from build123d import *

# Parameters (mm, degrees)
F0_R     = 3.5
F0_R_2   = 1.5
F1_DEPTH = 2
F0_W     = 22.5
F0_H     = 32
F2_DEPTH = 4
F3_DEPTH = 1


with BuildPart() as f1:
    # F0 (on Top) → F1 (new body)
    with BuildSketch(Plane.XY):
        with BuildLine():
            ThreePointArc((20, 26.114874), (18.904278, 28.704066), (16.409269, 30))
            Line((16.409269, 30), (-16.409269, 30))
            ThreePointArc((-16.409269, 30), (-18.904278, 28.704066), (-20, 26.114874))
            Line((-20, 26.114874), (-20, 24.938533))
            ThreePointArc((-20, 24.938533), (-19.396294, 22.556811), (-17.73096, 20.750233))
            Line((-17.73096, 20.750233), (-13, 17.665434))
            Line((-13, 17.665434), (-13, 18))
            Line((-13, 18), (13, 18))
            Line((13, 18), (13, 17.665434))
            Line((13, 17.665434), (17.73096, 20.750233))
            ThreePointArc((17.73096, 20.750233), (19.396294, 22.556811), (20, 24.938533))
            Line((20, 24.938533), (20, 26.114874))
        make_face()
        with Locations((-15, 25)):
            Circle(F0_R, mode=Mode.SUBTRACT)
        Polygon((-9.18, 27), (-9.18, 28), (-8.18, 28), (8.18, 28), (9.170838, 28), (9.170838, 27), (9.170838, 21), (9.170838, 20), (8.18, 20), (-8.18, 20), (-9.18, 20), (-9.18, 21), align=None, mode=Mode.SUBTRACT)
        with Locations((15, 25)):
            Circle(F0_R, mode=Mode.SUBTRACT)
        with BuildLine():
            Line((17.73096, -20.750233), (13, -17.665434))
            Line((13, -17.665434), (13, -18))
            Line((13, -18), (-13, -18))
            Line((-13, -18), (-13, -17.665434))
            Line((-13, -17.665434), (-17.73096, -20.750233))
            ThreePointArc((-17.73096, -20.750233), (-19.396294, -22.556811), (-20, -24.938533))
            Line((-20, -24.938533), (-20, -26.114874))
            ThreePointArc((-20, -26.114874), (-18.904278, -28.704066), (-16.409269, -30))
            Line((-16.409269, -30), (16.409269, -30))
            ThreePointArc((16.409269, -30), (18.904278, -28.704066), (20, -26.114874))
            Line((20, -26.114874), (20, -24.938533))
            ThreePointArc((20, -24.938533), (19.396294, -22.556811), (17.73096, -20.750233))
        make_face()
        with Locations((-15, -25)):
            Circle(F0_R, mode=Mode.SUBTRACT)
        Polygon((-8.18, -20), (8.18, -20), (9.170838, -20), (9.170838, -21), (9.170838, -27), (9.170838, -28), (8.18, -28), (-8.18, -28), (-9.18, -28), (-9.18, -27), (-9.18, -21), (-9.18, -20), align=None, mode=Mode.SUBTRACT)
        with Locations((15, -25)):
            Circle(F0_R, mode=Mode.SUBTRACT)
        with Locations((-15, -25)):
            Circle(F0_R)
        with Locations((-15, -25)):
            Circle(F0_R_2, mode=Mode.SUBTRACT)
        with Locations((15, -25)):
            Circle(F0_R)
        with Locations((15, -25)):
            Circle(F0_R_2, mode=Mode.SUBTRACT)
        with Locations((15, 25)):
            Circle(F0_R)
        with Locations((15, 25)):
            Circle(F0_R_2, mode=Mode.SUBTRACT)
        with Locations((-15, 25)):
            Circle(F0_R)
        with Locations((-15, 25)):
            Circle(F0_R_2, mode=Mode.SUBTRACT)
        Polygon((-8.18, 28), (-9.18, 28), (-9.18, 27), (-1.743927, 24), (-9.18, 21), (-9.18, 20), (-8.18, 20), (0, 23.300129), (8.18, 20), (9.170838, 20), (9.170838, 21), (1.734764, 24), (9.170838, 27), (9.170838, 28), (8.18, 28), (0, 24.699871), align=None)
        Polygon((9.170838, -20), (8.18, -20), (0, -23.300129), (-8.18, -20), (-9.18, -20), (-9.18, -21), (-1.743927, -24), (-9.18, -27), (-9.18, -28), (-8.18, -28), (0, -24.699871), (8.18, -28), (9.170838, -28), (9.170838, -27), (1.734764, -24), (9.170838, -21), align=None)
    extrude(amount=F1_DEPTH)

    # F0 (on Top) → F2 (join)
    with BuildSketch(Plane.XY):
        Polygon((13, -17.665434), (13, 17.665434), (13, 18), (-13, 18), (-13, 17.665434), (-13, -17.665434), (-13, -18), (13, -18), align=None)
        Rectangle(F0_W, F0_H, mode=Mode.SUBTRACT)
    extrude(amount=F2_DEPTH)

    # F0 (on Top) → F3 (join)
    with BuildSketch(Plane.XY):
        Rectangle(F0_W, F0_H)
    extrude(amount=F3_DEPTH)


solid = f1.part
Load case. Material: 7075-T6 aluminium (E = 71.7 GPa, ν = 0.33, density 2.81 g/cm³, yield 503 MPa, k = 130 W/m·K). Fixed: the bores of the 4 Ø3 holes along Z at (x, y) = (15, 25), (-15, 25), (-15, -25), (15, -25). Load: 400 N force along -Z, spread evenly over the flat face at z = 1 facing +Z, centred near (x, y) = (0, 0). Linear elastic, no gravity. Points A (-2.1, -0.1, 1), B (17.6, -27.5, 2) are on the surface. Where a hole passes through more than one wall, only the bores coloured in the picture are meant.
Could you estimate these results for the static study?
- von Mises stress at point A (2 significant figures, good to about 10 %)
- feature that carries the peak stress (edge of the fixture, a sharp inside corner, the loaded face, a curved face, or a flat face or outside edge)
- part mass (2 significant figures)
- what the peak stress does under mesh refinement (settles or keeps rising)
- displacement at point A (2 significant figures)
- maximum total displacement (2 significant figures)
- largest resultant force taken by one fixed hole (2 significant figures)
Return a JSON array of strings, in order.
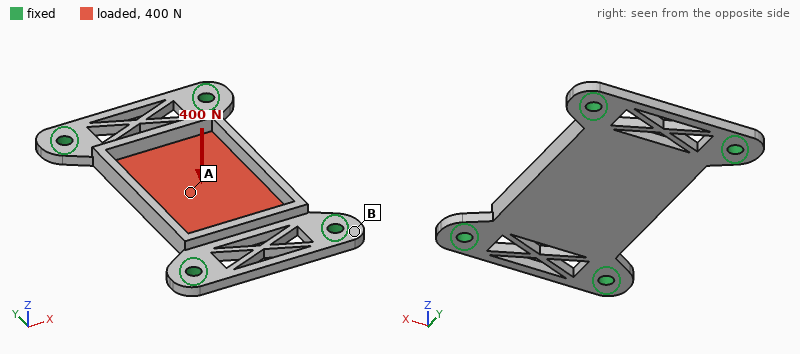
["75 MPa", "edge of the fixture", "8.2 g", "keeps rising", "0.21 mm", "0.22 mm", "100 N"]
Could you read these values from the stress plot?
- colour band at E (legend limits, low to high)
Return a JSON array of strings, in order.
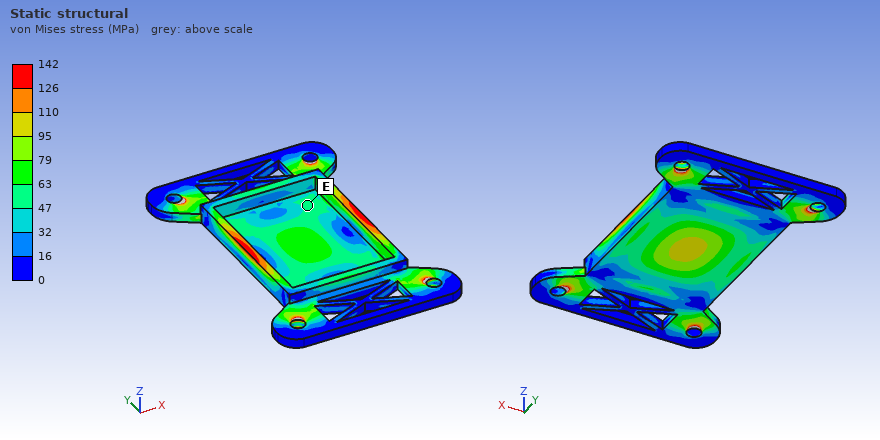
["47 to 63 MPa"]
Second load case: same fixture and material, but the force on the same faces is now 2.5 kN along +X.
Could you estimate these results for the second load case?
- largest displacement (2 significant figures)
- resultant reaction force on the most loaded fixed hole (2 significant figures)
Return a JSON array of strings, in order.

["55 µm", "820 N"]
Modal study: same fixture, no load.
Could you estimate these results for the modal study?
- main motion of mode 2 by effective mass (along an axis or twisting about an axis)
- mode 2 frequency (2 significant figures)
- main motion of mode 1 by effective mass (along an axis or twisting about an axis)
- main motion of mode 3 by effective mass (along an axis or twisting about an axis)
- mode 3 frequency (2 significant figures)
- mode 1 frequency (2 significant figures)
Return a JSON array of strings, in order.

["twisting about Y", "7600 Hz", "along Z", "twisting about X", "10 kHz", "4800 Hz"]
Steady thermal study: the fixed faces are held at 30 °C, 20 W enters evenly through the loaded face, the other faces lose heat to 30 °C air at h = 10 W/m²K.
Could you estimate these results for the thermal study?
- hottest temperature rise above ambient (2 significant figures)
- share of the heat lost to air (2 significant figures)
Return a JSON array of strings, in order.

["45 K", "3.8 %"]
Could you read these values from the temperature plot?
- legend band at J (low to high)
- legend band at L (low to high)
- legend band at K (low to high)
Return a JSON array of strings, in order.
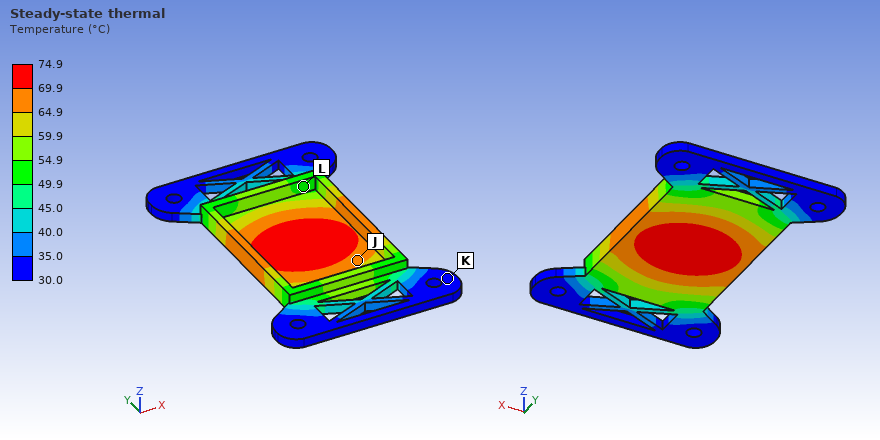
["64.9 to 69.9 °C", "49.9 to 54.9 °C", "30.0 to 35.0 °C"]
